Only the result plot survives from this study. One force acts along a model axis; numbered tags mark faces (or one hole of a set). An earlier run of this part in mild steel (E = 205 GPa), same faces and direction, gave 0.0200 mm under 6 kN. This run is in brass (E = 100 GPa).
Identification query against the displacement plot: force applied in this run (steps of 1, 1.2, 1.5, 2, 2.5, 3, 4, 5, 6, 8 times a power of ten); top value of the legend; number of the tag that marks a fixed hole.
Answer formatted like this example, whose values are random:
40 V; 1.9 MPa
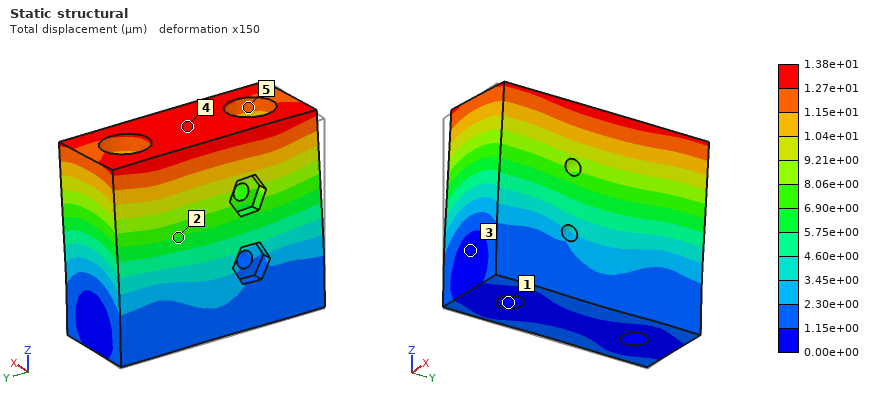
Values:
2 kN; 1.38e+01 µm; 1
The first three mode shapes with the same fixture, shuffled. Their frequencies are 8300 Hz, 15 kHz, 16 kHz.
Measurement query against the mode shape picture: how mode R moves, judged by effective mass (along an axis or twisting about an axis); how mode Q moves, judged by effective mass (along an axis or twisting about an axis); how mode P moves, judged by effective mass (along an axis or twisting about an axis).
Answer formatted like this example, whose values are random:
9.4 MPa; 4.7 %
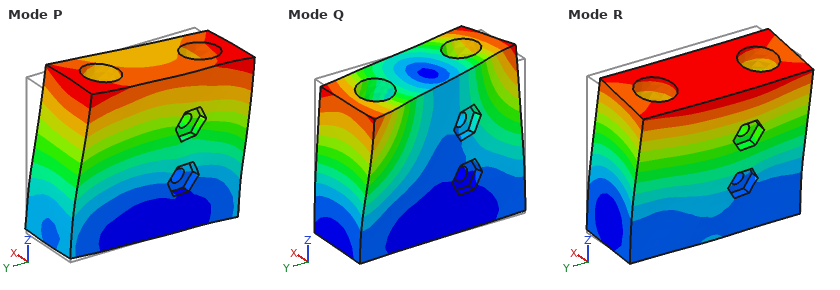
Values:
along X; twisting about Z; along Y
